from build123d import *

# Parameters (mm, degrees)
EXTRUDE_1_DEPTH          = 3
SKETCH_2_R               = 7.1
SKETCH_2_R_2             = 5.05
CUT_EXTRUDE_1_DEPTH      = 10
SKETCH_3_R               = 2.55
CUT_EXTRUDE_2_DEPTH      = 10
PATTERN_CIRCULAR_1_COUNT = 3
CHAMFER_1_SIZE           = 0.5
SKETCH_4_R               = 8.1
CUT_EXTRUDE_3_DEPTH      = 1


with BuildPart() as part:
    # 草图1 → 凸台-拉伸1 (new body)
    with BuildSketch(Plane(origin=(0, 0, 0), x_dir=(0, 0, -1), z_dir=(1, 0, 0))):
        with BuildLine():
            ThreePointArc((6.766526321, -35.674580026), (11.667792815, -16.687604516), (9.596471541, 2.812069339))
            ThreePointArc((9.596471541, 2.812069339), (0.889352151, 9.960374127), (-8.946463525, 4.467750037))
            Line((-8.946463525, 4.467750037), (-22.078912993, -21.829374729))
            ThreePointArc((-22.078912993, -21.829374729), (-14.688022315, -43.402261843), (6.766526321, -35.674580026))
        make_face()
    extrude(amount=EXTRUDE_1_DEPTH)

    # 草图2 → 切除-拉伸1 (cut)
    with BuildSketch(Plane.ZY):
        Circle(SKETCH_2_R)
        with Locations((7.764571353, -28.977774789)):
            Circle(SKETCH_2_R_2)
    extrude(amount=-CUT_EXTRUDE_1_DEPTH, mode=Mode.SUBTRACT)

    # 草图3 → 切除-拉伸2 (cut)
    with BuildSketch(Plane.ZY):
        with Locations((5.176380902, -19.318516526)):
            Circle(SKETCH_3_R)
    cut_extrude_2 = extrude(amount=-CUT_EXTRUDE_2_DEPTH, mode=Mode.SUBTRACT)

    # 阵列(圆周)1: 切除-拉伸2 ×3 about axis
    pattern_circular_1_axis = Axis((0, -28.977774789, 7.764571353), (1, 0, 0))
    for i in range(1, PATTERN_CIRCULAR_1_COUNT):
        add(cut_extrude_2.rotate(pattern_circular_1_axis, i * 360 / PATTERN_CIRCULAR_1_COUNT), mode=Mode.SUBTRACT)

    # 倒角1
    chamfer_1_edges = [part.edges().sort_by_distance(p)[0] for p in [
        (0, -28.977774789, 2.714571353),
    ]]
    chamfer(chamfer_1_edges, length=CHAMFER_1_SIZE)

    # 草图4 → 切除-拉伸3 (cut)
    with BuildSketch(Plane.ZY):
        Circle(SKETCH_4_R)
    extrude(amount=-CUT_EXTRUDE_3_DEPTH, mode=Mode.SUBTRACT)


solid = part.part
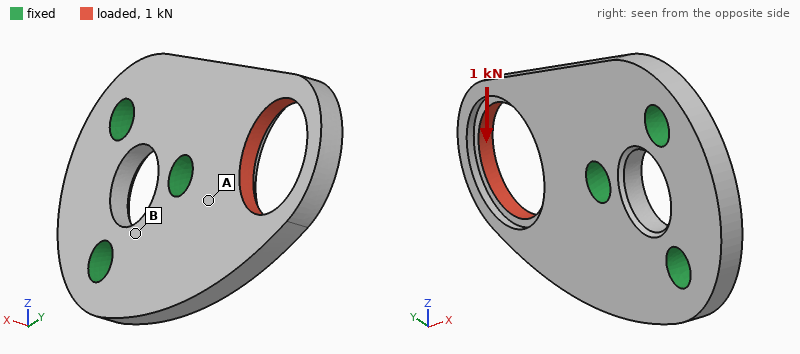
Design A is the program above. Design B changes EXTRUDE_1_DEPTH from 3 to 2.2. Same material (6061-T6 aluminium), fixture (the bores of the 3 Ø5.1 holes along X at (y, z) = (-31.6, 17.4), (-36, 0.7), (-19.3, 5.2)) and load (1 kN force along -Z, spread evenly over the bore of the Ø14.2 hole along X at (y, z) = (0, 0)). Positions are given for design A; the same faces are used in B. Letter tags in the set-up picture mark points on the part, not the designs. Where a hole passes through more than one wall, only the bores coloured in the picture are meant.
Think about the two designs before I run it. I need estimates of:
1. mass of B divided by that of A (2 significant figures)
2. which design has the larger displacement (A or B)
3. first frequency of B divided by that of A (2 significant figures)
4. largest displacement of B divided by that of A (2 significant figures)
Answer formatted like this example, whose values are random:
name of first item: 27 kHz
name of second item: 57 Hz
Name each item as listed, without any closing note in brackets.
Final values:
mass of B divided by that of A: 0.73
which design has the larger displacement: B
first frequency of B divided by that of A: 0.76
largest displacement of B divided by that of A: 1.5
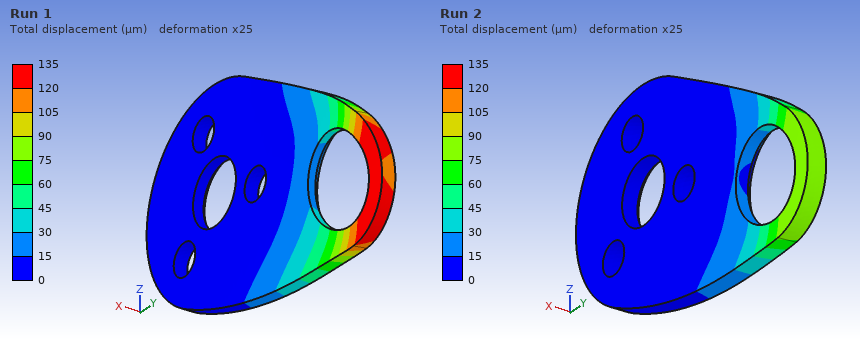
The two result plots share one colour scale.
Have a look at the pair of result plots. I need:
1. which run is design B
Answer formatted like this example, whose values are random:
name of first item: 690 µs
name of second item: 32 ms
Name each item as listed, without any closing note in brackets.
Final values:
which run is design B: Run 1
